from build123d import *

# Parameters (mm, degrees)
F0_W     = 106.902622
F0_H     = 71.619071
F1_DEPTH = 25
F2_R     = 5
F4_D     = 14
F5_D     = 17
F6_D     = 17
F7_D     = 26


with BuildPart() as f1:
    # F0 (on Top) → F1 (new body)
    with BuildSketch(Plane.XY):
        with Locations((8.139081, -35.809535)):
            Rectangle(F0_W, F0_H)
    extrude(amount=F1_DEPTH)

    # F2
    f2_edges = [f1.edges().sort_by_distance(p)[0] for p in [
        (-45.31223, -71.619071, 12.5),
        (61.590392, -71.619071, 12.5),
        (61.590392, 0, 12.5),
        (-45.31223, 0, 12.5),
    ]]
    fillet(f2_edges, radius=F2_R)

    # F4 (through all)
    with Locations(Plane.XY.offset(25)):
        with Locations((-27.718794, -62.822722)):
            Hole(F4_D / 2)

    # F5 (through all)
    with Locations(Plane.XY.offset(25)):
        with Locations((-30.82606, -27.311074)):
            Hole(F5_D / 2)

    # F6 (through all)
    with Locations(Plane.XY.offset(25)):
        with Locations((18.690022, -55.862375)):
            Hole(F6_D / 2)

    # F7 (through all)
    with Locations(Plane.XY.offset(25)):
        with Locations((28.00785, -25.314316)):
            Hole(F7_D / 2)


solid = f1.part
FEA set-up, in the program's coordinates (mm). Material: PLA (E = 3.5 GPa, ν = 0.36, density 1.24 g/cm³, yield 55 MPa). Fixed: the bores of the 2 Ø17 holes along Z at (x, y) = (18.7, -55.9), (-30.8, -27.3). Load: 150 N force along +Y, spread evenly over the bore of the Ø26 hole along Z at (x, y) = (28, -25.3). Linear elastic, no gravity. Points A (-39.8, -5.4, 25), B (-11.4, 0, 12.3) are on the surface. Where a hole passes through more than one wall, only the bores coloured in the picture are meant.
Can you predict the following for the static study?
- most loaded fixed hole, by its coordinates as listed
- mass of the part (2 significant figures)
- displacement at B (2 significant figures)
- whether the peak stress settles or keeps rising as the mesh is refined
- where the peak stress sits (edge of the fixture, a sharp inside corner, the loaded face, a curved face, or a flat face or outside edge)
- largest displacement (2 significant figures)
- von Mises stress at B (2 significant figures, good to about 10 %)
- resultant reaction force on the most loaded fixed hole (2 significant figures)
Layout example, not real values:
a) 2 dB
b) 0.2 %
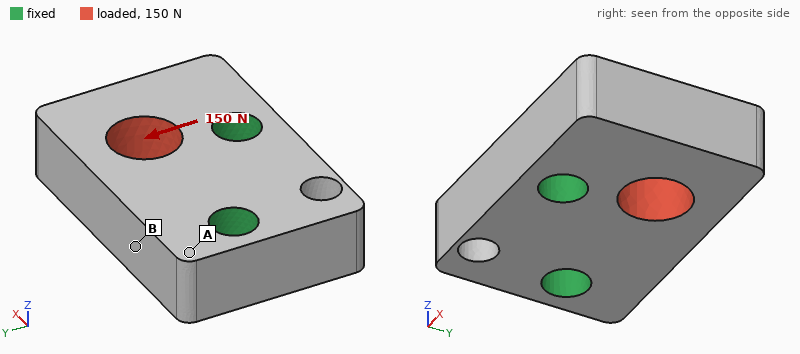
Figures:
a) (18.7, -55.9)
b) 200 g
c) 0.88 µm
d) keeps rising
e) edge of the fixture
f) 4.0 µm
g) 0.084 MPa
h) 150 N
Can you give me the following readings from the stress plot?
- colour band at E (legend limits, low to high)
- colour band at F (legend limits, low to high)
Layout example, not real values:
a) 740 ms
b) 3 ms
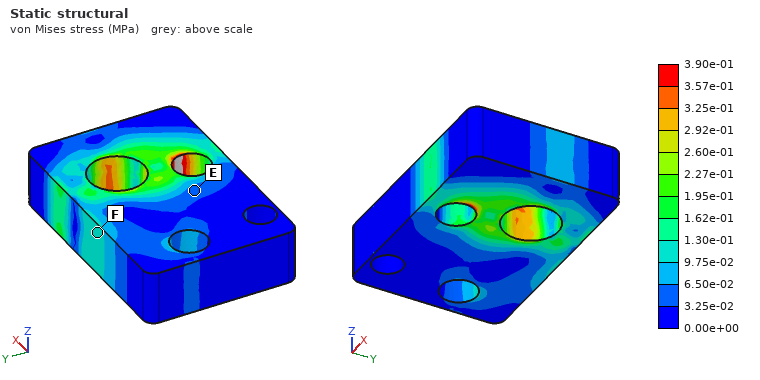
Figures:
a) 3.25e-02 to 6.50e-02 MPa
b) 9.75e-02 to 1.30e-01 MPa
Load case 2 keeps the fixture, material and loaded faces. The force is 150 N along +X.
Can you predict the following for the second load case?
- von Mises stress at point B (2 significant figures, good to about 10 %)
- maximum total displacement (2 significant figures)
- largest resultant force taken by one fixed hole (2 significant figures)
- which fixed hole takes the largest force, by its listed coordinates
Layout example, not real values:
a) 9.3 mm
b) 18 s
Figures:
a) 0.092 MPa
b) 3.1 µm
c) 85 N
d) (-30.8, -27.3)
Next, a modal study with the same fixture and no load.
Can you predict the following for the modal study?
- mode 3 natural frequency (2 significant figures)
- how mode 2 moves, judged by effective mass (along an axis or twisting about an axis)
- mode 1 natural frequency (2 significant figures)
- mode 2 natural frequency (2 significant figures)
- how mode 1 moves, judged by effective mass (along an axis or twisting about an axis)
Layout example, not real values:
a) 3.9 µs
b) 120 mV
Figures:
a) 3500 Hz
b) along Y
c) 1800 Hz
d) 3100 Hz
e) along Z
